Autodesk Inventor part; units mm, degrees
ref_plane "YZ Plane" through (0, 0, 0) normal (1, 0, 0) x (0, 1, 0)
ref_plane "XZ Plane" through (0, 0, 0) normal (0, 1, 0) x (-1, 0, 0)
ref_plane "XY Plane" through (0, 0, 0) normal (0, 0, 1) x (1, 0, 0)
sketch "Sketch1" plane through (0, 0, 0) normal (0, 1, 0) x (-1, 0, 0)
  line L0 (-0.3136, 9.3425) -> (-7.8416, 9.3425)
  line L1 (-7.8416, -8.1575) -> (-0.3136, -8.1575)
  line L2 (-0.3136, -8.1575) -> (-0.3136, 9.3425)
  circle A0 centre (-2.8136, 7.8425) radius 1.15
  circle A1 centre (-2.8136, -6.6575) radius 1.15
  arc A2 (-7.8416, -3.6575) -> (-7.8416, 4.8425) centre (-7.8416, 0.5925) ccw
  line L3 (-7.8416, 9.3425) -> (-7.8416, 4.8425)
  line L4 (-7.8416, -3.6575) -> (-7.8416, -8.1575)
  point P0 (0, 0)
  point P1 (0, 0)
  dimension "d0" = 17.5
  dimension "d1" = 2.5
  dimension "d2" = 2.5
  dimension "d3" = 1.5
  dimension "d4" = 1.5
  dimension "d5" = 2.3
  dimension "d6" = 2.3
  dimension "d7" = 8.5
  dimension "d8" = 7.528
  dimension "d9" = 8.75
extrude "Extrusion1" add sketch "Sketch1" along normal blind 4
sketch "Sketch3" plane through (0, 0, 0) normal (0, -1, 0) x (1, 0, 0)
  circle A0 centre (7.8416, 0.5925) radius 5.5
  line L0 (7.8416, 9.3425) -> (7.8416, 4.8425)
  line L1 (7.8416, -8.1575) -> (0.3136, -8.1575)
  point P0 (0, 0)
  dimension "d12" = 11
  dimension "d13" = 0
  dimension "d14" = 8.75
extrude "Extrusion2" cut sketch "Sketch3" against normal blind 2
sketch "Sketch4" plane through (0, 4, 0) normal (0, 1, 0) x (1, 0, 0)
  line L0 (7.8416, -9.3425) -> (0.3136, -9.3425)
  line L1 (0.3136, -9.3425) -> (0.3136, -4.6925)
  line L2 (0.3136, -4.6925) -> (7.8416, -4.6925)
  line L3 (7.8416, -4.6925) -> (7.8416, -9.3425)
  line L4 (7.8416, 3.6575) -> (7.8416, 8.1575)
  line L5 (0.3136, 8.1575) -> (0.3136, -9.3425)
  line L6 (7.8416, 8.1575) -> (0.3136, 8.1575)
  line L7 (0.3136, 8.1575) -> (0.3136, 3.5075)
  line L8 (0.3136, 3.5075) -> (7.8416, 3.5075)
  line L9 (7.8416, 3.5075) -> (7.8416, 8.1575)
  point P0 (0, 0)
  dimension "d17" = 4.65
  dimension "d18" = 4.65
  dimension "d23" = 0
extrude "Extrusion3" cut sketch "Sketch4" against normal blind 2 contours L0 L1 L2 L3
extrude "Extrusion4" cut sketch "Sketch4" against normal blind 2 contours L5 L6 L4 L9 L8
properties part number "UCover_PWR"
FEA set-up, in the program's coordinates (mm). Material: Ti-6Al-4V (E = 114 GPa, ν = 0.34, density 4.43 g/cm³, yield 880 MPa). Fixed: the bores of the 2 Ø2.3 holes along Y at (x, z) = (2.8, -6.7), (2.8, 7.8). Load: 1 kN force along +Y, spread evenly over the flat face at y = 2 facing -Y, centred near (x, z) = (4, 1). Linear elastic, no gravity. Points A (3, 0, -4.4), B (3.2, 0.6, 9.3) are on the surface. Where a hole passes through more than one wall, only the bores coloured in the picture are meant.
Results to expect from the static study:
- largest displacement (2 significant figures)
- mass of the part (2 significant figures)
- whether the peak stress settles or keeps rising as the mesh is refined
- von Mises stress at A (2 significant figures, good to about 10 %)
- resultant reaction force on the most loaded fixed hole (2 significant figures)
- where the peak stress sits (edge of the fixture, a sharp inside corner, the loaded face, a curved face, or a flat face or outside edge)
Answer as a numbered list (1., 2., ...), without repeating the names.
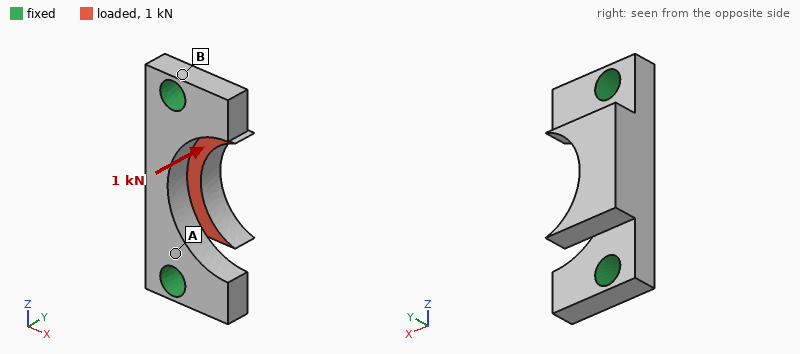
1. 46 µm
2. 0.97 g
3. keeps rising
4. 210 MPa
5. 590 N
6. a sharp inside corner
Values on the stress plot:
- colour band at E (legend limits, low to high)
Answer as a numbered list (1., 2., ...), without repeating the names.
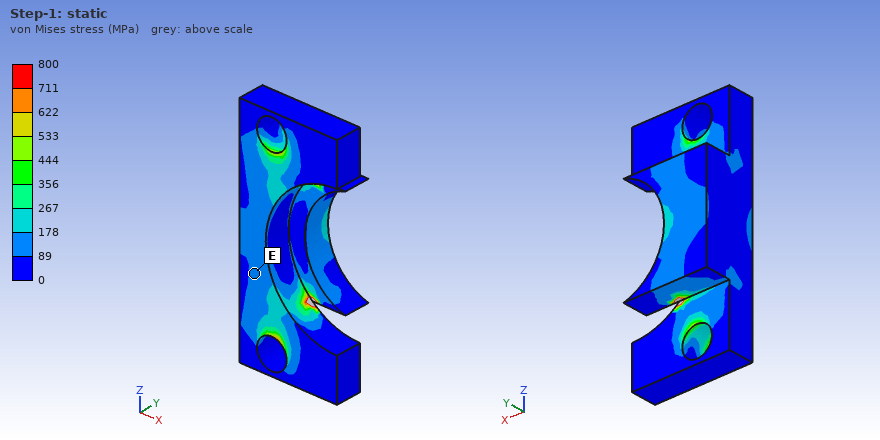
1. 89 to 178 MPa
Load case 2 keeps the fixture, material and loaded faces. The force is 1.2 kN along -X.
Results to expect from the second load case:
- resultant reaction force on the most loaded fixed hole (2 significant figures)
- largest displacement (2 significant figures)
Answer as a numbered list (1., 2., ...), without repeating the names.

1. 650 N
2. 29 µm
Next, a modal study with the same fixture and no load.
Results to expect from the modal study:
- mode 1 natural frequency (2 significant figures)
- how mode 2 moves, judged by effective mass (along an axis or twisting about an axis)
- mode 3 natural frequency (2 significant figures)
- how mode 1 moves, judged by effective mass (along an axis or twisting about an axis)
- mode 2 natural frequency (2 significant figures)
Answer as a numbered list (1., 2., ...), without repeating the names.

1. 47 kHz
2. along Y
3. 83 kHz
4. along X
5. 64 kHz
